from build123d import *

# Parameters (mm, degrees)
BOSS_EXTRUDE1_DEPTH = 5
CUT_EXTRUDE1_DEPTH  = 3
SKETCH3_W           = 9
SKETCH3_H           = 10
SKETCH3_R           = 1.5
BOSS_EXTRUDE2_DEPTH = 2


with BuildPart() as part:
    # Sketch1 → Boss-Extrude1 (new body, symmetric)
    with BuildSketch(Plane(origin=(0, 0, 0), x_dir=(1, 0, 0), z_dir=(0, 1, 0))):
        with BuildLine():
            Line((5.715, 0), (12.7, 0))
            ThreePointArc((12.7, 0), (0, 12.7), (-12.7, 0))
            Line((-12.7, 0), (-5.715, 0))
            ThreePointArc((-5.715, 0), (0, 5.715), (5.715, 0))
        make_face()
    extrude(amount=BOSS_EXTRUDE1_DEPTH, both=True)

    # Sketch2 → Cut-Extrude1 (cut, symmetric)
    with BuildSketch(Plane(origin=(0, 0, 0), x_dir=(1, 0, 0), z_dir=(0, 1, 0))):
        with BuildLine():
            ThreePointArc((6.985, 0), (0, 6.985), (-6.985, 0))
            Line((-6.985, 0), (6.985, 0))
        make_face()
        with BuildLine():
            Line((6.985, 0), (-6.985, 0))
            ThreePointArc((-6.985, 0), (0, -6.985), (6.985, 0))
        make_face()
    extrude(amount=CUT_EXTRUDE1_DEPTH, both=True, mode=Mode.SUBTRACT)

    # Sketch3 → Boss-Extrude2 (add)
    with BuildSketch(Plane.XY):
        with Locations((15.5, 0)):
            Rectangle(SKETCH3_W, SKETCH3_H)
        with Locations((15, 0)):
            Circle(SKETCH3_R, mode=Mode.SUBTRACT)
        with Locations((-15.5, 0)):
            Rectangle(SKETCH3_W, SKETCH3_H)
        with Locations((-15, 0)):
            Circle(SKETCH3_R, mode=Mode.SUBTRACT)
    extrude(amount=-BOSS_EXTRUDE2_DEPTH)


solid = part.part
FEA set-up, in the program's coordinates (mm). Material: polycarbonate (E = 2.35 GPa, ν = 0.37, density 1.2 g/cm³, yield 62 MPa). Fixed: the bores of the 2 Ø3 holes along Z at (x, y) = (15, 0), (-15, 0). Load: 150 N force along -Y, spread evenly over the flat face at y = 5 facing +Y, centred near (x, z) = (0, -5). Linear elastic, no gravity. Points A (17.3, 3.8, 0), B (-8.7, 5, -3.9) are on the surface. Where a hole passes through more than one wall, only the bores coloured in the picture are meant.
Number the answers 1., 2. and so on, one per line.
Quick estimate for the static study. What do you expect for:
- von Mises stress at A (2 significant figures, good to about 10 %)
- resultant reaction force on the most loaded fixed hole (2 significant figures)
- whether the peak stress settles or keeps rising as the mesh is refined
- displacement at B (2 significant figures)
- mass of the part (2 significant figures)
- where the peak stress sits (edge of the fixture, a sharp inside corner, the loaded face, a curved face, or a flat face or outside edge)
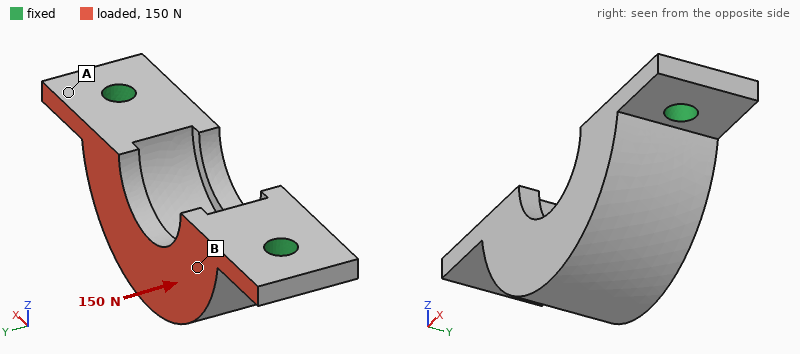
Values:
1. 9.7 MPa
2. 75 N
3. keeps rising
4. 0.18 mm
5. 2.6 g
6. edge of the fixture
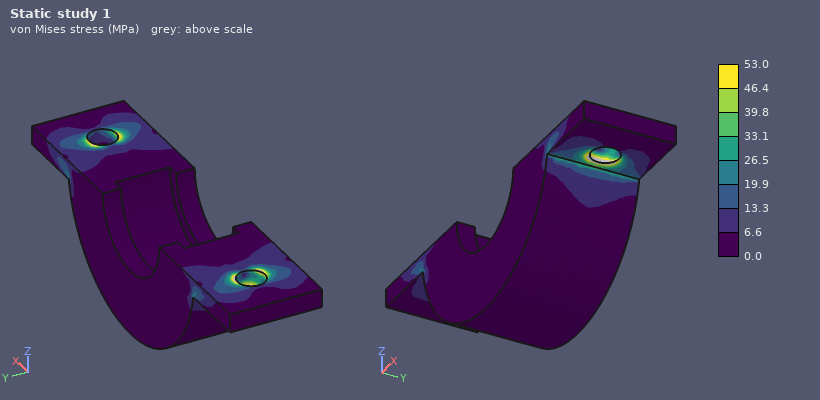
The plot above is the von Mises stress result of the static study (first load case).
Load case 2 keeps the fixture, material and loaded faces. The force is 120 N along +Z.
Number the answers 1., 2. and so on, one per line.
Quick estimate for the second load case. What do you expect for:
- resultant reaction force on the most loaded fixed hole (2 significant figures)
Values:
1. 73 N
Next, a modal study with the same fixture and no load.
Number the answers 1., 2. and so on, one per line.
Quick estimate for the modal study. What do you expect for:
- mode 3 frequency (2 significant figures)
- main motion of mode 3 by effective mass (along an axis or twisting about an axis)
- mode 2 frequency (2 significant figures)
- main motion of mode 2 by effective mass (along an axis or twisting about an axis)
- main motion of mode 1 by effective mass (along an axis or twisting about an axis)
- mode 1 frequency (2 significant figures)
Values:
1. 9500 Hz
2. along X
3. 6800 Hz
4. along Z
5. along Y
6. 2300 Hz
